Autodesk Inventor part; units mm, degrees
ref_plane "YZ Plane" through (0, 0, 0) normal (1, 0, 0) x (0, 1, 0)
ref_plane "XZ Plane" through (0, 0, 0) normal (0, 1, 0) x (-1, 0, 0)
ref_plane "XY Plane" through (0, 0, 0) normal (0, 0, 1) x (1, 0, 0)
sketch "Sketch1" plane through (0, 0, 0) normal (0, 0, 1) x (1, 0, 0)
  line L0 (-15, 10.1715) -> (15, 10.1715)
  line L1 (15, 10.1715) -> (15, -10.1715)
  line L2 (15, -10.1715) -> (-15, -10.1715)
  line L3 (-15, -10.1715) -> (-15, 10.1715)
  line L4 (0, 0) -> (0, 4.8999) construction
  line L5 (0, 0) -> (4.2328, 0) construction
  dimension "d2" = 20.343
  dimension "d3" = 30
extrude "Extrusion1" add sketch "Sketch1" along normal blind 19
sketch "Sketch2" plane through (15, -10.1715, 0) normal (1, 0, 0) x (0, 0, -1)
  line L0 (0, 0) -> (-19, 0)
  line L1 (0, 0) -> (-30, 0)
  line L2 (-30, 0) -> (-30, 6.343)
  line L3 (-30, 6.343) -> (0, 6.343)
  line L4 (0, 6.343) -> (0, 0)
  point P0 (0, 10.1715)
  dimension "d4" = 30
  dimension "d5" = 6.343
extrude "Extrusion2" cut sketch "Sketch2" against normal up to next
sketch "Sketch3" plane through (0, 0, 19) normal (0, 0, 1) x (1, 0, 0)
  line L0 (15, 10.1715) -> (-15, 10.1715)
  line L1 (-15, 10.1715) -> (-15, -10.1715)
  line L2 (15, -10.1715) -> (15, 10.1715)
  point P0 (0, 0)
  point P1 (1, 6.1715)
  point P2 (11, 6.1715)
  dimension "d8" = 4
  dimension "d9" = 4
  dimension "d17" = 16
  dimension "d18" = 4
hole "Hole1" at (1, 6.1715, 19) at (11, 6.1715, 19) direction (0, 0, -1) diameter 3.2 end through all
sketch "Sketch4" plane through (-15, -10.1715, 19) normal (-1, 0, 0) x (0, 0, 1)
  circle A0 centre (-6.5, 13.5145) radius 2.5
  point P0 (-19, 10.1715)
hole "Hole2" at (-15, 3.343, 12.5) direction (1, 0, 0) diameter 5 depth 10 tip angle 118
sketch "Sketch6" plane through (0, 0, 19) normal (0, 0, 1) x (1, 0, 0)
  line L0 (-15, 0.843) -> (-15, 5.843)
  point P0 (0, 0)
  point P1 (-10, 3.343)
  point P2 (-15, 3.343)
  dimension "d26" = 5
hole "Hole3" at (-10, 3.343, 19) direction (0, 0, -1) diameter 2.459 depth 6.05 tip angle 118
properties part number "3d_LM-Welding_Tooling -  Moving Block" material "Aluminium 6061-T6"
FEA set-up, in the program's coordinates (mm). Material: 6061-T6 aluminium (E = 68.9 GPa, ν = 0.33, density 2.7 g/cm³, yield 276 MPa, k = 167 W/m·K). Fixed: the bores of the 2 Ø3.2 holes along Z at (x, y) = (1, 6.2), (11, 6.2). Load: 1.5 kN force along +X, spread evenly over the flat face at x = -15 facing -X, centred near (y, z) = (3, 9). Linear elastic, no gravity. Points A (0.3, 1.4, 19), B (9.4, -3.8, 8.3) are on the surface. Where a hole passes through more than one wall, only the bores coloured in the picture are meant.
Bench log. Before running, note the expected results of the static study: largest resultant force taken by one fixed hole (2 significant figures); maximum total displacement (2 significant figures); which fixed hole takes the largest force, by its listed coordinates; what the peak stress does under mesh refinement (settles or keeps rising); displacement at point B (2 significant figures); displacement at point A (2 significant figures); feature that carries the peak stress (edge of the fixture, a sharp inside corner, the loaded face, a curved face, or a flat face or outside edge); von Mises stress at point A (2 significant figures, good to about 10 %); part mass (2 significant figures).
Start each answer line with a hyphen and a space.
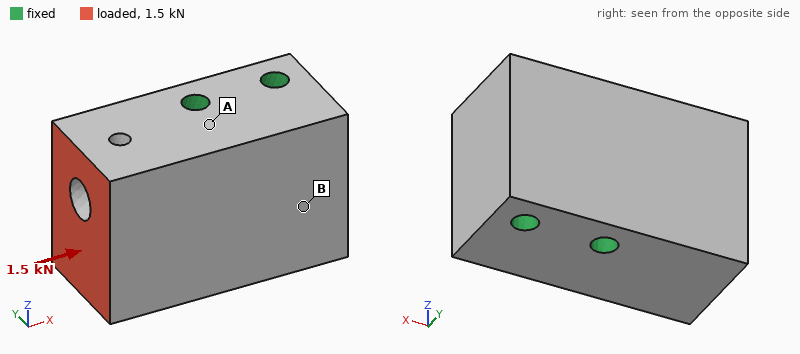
- 1.2 kN
- 3.1 µm
- (1, 6.2)
- keeps rising
- 0.66 µm
- 0.70 µm
- edge of the fixture
- 5.0 MPa
- 20 g
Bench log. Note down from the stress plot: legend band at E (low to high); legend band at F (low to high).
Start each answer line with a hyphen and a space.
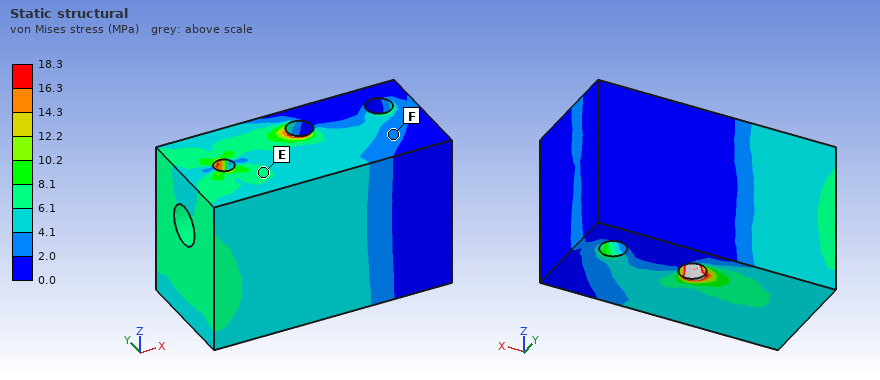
- 6.1 to 8.1 MPa
- 2.0 to 4.1 MPa
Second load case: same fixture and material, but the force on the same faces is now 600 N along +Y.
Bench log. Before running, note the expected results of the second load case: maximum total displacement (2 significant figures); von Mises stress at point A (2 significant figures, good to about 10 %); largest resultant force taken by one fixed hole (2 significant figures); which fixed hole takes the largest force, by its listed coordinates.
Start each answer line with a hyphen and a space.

- 8.6 µm
- 5.4 MPa
- 1.2 kN
- (1, 6.2)
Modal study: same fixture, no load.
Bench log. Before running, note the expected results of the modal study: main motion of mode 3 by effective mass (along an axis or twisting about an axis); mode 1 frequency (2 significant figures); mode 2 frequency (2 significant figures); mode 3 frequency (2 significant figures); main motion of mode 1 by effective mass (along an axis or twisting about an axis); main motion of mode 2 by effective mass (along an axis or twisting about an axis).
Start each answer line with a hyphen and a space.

- twisting about X
- 23 kHz
- 32 kHz
- 41 kHz
- along Y
- along Z
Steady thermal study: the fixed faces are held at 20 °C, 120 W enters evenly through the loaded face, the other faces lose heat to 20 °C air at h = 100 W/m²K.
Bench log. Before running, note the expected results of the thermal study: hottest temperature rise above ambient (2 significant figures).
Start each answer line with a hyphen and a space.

- 48 K
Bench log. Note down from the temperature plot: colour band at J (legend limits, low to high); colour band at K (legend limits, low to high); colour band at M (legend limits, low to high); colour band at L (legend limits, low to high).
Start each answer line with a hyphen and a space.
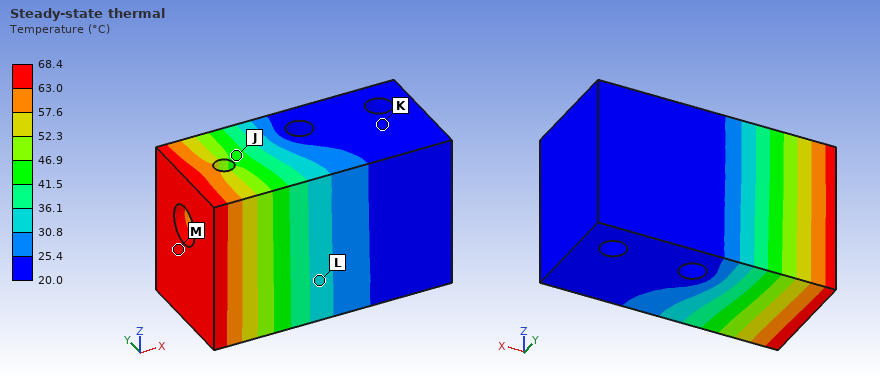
- 41.5 to 46.9 °C
- 20.0 to 25.4 °C
- 63.0 to 68.4 °C
- 30.8 to 36.1 °C
